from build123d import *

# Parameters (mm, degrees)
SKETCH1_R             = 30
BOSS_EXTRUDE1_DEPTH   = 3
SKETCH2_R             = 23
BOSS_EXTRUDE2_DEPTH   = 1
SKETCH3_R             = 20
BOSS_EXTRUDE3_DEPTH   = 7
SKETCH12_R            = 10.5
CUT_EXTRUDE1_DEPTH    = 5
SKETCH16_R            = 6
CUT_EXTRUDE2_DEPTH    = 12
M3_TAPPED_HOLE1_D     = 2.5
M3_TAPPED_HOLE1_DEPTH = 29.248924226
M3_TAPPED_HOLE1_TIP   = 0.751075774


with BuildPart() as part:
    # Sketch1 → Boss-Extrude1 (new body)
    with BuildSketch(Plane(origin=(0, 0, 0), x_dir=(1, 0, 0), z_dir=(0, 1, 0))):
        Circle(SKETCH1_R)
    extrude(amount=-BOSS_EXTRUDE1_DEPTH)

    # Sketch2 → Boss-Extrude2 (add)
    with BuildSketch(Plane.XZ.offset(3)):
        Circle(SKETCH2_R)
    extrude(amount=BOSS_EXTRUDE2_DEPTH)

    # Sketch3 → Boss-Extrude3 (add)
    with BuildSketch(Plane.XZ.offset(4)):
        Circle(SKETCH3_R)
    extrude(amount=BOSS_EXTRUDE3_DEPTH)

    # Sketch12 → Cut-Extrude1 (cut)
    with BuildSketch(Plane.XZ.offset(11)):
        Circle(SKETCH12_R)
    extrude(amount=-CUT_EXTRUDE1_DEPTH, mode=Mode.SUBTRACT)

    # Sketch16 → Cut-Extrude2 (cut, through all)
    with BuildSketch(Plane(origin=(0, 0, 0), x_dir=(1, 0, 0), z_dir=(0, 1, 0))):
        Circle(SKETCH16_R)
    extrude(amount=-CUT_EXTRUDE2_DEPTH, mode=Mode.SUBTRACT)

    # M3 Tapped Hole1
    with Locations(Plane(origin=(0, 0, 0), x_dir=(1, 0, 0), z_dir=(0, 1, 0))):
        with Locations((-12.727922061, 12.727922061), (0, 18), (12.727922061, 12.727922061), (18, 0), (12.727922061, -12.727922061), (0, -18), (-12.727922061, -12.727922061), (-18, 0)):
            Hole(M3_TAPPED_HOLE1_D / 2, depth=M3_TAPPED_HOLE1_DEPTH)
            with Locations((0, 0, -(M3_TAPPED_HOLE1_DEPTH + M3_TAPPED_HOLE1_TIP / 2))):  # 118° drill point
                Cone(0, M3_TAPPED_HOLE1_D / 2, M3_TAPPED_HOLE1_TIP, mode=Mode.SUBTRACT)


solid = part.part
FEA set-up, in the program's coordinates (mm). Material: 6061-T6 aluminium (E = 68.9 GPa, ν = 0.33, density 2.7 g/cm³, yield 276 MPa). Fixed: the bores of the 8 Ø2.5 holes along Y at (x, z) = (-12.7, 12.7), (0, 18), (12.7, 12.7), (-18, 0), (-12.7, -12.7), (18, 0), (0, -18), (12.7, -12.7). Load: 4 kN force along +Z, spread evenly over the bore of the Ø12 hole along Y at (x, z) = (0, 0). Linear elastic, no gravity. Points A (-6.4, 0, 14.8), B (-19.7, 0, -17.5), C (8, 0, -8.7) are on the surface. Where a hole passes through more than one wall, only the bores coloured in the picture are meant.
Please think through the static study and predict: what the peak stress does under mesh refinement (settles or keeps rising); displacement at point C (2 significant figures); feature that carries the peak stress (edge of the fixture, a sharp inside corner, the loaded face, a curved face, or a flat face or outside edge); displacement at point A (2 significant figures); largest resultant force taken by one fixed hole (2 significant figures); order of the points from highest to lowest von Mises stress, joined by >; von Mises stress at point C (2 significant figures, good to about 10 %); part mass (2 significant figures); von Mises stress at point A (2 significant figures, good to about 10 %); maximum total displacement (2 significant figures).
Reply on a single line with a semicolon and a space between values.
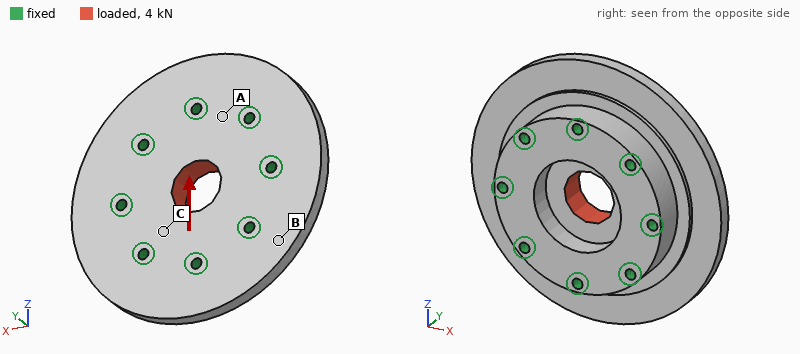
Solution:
keeps rising; 1.2 µm; edge of the fixture; 0.95 µm; 810 N; C > A > B; 12 MPa; 43 g; 5.9 MPa; 3.0 µm
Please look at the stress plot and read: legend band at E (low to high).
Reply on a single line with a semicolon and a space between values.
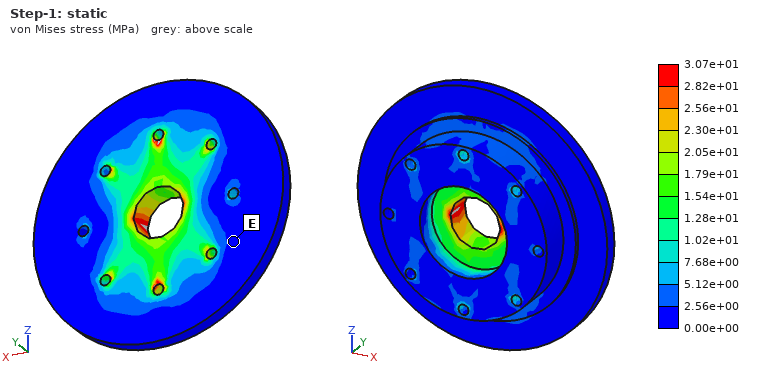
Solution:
0.00e+00 to 2.56e+00 MPa
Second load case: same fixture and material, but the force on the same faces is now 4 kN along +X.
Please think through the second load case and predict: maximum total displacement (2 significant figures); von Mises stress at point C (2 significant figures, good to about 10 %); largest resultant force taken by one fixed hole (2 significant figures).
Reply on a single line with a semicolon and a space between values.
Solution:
3.0 µm; 11 MPa; 810 N
